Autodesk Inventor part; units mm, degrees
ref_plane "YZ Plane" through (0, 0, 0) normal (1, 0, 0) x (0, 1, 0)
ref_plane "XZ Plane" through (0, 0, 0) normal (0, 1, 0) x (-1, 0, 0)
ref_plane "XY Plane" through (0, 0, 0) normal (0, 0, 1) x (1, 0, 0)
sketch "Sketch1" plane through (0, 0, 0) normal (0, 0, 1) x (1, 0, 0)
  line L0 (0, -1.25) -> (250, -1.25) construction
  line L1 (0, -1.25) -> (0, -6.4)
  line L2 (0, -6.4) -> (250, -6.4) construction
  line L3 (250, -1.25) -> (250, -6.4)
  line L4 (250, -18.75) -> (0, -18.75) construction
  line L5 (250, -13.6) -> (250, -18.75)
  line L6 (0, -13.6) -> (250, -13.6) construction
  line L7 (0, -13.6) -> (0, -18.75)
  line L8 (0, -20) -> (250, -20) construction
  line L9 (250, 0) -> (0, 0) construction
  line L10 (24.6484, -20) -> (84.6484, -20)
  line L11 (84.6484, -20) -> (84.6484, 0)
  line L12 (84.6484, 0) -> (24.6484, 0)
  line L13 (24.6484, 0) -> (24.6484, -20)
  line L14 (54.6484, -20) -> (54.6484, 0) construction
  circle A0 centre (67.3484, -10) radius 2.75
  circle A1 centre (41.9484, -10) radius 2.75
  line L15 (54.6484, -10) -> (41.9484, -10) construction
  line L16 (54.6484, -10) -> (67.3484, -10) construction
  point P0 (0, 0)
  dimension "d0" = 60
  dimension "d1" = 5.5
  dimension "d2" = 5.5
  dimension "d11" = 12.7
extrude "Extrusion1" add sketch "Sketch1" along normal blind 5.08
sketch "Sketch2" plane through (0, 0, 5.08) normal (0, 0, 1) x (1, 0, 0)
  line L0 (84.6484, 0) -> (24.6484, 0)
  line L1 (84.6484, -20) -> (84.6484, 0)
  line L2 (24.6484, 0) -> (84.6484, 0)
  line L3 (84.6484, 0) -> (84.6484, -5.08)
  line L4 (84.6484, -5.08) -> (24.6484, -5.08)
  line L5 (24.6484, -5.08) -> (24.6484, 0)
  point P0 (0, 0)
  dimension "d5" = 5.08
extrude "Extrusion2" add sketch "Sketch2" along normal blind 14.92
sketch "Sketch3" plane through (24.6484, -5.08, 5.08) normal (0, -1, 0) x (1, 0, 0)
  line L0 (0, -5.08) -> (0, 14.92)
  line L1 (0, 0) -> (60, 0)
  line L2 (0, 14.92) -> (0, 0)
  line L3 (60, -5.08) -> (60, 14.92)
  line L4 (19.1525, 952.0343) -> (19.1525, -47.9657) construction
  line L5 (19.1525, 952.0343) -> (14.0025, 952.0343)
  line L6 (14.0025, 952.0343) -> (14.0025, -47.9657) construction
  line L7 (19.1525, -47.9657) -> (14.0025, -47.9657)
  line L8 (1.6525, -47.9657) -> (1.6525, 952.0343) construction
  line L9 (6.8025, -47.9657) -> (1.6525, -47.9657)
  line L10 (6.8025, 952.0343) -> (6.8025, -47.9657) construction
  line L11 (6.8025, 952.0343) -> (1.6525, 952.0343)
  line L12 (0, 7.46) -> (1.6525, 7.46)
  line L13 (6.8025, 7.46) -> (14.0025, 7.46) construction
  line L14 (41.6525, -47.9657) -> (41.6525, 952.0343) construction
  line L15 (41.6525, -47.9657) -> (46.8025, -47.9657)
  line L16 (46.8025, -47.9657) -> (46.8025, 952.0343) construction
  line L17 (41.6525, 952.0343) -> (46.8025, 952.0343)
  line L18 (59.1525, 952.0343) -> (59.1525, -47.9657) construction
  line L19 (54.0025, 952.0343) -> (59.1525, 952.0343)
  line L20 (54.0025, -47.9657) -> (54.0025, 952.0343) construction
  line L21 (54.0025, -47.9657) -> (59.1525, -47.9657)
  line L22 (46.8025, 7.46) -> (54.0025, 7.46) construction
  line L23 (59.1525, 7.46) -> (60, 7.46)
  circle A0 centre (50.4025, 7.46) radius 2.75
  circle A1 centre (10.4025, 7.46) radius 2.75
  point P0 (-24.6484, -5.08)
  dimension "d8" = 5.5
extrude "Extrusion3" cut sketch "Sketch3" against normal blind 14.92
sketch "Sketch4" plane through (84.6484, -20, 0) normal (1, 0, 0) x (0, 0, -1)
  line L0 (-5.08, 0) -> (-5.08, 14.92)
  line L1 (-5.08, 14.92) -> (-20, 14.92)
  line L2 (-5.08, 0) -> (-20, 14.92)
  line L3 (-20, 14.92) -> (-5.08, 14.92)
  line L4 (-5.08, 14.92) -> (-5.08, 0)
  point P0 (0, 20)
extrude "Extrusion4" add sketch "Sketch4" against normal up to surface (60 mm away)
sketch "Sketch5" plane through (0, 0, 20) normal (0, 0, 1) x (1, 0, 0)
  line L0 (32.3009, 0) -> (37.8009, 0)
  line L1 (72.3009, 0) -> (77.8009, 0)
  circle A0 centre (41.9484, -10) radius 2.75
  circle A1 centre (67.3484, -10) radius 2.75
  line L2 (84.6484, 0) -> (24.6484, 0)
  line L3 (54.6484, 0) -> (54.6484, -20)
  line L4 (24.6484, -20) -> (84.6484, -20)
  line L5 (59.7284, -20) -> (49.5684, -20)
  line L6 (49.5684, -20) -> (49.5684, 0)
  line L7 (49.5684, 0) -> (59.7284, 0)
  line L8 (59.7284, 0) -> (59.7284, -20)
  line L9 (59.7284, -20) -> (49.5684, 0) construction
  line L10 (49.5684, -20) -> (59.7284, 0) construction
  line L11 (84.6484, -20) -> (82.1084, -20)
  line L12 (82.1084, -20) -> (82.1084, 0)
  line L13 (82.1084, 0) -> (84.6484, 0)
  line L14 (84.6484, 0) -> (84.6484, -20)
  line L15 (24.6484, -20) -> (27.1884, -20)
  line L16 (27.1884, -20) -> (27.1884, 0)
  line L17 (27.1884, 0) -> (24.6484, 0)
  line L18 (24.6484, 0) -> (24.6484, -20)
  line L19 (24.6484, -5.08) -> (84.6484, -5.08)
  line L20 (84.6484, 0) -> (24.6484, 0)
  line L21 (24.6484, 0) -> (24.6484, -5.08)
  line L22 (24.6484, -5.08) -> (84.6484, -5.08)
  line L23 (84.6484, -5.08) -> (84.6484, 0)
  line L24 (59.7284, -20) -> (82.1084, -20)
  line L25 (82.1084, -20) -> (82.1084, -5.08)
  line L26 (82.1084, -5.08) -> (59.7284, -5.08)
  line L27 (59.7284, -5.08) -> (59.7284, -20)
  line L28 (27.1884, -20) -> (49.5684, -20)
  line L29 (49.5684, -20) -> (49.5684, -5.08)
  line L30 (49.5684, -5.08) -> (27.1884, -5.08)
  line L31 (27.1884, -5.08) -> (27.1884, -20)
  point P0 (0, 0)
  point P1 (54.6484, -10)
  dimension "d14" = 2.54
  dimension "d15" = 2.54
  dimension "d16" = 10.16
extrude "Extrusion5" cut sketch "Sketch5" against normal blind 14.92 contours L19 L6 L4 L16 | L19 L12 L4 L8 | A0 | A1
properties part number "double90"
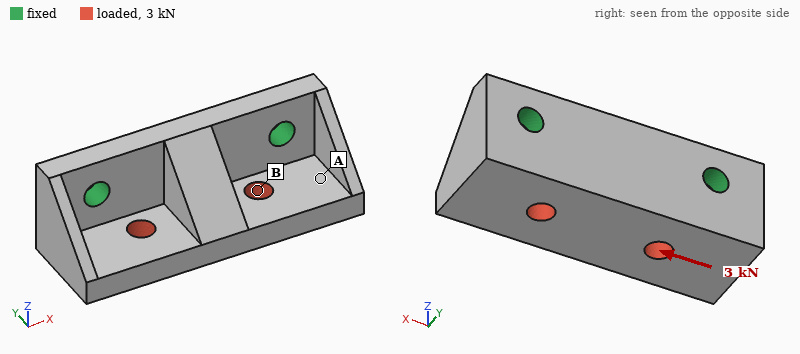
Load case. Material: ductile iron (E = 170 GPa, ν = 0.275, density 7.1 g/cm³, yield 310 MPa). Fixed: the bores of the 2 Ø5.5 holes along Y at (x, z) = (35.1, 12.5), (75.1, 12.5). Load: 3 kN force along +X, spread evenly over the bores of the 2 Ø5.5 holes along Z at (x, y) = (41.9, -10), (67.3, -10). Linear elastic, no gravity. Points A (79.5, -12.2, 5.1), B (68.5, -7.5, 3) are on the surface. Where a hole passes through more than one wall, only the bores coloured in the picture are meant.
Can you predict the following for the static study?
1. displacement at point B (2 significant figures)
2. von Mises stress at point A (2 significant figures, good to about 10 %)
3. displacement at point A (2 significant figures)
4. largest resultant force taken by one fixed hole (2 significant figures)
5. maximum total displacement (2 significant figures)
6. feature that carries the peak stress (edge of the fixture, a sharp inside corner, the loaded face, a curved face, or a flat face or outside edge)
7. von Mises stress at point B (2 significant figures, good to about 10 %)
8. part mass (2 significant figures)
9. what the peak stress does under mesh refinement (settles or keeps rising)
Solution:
3.1 µm
12 MPa
4.5 µm
1.7 kN
7.0 µm
edge of the fixture
38 MPa
84 g
keeps rising
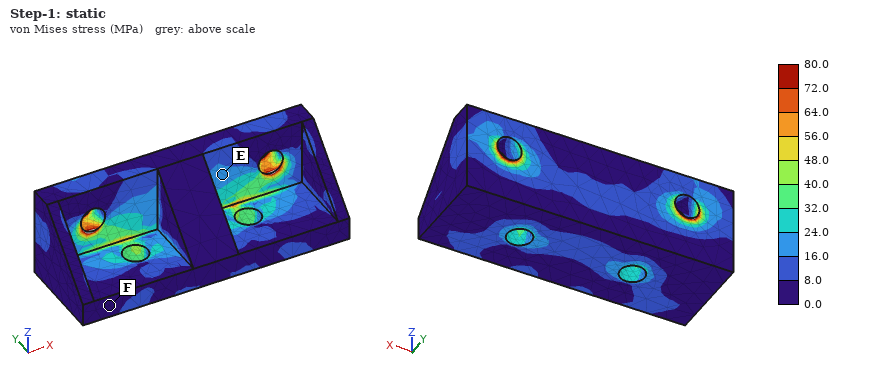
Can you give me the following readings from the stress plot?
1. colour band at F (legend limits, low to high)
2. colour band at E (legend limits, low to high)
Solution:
0.0 to 8.0 MPa
16.0 to 24.0 MPa
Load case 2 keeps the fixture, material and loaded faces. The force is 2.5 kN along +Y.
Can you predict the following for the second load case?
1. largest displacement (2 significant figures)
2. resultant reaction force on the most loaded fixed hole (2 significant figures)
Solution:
23 µm
1.3 kN
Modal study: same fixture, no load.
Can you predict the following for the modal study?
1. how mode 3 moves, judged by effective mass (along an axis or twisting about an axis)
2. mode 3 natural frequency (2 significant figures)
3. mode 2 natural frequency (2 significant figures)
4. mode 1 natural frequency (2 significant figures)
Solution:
along Y
14 kHz
12 kHz
7700 Hz
